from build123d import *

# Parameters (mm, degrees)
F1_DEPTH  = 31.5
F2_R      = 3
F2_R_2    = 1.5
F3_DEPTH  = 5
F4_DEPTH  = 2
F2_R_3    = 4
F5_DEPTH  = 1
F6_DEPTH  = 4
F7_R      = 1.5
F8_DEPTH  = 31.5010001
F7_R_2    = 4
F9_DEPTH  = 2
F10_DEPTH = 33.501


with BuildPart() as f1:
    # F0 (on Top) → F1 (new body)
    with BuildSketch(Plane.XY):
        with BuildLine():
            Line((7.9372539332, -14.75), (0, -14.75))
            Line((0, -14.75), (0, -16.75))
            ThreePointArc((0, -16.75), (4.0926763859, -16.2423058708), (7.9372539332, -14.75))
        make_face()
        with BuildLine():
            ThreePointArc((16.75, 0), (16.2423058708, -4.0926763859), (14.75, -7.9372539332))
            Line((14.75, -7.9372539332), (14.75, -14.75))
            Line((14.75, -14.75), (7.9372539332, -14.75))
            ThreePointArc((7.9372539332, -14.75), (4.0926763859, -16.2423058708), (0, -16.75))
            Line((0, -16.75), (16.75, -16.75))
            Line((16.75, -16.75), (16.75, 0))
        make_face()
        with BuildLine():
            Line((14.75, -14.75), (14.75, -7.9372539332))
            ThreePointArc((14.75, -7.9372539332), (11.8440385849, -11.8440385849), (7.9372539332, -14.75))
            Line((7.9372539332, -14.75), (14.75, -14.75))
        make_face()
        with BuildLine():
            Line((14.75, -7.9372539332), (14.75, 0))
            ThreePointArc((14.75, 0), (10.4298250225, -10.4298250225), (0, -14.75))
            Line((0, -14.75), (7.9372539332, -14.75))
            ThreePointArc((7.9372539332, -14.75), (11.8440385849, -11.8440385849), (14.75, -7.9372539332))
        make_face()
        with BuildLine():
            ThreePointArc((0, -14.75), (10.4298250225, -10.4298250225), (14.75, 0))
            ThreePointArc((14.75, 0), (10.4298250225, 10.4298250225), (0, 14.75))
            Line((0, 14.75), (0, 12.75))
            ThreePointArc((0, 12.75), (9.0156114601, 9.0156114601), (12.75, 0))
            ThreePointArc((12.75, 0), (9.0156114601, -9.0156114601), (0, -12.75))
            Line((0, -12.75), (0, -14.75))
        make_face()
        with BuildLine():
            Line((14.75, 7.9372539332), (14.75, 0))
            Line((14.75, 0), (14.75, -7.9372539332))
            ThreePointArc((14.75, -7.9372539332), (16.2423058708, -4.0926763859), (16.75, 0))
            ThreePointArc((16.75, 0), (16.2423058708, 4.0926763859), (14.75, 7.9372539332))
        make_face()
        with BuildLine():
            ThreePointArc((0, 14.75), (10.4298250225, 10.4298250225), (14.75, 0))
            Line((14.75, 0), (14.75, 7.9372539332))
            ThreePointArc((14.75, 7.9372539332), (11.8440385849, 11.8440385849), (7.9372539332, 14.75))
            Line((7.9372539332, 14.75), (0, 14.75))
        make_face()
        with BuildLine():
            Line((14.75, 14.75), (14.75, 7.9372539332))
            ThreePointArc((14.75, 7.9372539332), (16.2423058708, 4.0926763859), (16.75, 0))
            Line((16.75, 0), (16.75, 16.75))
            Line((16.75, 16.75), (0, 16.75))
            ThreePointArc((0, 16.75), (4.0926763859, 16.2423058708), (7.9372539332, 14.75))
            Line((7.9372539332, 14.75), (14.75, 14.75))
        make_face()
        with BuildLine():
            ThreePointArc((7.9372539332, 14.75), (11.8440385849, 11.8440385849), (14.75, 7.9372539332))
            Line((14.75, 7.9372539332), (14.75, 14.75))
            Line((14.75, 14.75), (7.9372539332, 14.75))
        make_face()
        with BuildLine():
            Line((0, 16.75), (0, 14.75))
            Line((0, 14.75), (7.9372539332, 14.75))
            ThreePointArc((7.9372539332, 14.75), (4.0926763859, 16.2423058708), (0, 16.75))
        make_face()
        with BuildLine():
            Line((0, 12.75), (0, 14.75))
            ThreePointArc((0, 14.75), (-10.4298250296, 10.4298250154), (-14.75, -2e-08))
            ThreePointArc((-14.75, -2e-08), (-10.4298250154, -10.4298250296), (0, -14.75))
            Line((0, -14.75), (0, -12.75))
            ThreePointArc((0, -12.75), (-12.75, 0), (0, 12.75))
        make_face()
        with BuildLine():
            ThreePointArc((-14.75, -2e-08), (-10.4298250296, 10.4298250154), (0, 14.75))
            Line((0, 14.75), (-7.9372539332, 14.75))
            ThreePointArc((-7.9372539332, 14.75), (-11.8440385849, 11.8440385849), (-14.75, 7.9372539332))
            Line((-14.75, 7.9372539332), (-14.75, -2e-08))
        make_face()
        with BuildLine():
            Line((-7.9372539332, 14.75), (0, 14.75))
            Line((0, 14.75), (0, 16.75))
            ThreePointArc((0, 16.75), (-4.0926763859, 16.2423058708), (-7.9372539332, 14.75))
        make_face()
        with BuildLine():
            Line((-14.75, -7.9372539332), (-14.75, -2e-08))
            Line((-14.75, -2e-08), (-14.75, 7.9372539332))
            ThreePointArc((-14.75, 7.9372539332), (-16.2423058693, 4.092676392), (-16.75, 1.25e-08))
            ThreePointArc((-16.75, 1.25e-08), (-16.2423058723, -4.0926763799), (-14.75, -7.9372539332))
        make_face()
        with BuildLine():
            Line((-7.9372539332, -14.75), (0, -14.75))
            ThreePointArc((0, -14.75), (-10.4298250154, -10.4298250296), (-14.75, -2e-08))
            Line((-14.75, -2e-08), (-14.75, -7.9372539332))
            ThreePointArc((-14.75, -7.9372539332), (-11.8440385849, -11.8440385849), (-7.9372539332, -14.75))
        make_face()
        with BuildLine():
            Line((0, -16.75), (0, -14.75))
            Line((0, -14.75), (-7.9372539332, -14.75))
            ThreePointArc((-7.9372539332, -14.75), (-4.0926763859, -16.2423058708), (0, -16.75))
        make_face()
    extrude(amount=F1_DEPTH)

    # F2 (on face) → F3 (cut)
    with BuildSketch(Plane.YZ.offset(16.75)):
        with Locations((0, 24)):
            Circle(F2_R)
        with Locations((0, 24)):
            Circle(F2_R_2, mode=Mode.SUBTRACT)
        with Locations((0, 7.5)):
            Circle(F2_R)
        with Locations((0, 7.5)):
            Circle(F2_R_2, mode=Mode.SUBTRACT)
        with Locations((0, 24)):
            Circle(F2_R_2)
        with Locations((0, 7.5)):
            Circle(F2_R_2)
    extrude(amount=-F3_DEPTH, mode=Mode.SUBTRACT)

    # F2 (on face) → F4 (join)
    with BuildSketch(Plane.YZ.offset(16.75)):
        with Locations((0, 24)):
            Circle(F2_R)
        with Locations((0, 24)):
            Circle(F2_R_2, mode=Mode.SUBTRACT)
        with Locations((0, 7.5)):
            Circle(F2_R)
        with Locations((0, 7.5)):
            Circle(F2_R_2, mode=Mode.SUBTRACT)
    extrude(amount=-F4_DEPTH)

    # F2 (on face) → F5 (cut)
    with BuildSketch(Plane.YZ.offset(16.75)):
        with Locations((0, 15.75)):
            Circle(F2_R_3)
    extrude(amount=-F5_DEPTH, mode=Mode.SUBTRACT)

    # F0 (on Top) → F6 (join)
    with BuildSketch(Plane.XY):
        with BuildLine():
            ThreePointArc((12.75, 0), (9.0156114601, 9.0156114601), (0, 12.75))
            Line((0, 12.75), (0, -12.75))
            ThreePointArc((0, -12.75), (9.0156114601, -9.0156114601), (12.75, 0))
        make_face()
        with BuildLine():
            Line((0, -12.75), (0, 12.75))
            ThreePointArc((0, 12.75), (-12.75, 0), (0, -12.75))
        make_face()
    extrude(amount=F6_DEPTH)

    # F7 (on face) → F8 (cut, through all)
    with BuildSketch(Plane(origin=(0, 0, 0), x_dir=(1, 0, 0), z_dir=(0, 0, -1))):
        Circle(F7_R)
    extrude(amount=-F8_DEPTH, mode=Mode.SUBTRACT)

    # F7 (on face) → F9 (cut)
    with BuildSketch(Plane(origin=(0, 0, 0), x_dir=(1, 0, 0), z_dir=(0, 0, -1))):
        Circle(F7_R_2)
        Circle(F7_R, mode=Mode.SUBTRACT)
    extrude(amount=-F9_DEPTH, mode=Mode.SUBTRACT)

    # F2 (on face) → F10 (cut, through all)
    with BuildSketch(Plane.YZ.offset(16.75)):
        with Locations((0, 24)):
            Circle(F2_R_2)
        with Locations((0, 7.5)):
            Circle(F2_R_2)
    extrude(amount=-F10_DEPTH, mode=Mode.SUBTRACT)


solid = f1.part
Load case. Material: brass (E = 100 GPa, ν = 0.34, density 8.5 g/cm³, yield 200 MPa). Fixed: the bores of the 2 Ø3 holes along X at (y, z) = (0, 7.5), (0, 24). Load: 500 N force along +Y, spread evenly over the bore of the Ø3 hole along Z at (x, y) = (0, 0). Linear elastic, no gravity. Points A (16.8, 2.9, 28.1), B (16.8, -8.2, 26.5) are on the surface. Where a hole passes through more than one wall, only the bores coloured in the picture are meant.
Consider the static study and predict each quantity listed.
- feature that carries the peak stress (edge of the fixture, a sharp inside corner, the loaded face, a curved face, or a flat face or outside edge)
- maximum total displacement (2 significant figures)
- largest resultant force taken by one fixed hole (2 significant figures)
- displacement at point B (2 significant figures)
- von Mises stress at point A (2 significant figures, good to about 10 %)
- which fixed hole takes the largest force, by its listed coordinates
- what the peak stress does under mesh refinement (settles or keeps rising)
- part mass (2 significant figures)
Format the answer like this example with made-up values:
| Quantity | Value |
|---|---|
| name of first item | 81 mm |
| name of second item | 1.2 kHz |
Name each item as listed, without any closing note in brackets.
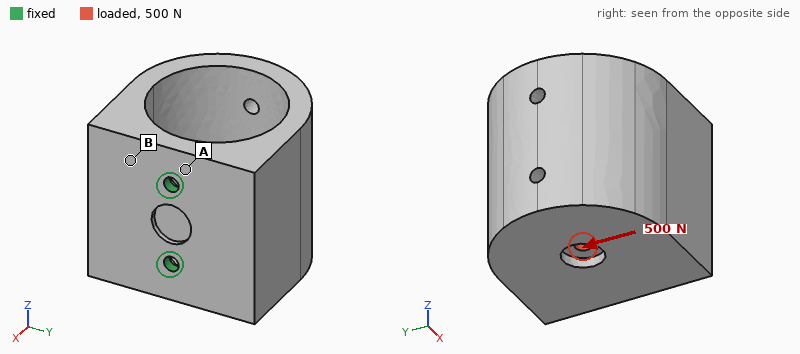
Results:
| Quantity | Value |
|---|---|
| feature that carries the peak stress | edge of the fixture |
| maximum total displacement | 0.13 mm |
| largest resultant force taken by one fixed hole | 600 N |
| displacement at point B | 0.029 mm |
| von Mises stress at point A | 39 MPa |
| which fixed hole takes the largest force, by its listed coordinates | (0, 7.5) |
| what the peak stress does under mesh refinement | keeps rising |
| part mass | 150 g |
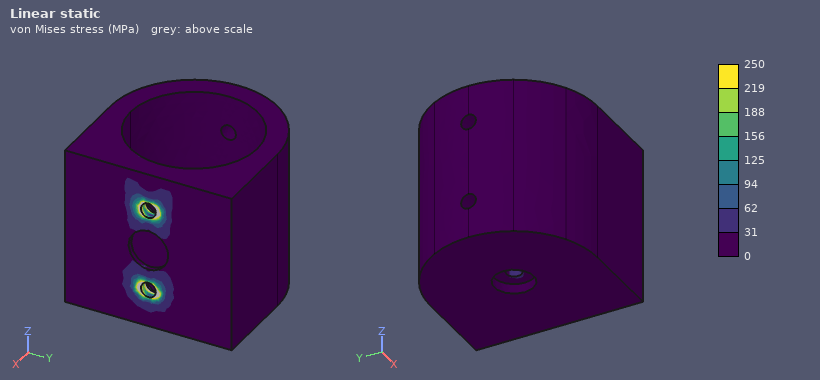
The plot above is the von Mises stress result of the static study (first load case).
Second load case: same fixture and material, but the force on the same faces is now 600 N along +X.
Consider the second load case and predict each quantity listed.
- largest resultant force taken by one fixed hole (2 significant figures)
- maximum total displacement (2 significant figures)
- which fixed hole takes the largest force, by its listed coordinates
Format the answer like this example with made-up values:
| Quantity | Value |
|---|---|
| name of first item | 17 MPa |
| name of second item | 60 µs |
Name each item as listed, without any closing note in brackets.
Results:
| Quantity | Value |
|---|---|
| largest resultant force taken by one fixed hole | 720 N |
| maximum total displacement | 11 µm |
| which fixed hole takes the largest force, by its listed coordinates | (0, 7.5) |
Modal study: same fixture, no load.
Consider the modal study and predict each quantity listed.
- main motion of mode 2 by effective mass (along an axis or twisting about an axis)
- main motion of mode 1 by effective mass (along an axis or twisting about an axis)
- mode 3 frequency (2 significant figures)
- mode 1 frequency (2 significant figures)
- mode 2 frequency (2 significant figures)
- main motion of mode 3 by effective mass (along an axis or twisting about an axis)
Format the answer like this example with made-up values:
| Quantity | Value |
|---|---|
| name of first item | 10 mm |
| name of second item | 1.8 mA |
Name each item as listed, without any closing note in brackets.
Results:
| Quantity | Value |
|---|---|
| main motion of mode 2 by effective mass | along Z |
| main motion of mode 1 by effective mass | along Y |
| mode 3 frequency | 5700 Hz |
| mode 1 frequency | 940 Hz |
| mode 2 frequency | 2900 Hz |
| main motion of mode 3 by effective mass | along X |
